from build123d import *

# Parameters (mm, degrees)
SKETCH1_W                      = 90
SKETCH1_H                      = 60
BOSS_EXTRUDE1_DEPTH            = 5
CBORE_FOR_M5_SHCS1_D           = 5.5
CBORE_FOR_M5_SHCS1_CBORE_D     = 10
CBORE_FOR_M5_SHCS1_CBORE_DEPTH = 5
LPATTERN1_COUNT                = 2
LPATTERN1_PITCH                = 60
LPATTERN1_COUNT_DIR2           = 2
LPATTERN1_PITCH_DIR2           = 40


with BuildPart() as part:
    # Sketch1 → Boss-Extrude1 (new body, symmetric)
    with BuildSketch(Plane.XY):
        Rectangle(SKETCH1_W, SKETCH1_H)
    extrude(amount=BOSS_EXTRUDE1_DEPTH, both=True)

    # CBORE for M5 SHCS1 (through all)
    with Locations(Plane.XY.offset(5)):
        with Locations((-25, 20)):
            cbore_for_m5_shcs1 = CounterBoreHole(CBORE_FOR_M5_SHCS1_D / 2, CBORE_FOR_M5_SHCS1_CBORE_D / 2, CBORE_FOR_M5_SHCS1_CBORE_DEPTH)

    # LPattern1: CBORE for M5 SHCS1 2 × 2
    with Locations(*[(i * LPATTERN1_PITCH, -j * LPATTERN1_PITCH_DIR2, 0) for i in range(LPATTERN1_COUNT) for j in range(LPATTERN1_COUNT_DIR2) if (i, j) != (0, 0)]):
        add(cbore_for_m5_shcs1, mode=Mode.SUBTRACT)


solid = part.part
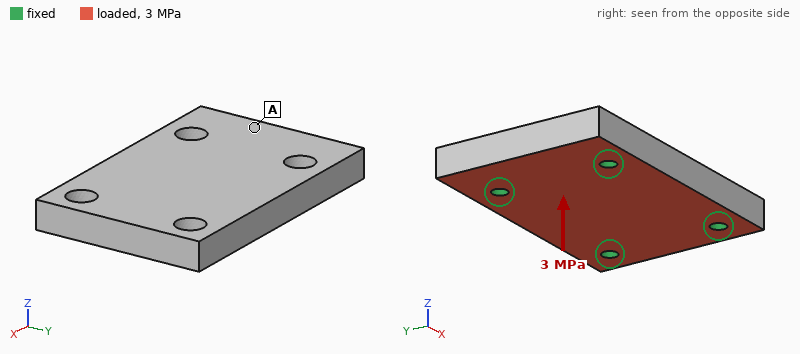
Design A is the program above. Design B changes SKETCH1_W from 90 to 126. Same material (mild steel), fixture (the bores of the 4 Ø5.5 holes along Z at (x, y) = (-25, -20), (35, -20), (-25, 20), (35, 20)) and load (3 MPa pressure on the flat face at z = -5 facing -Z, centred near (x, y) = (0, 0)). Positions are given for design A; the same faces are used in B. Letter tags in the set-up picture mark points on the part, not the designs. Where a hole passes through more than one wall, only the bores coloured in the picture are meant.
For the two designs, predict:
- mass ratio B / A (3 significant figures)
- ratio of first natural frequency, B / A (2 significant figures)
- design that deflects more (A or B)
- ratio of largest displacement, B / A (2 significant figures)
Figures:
1.42
0.46
B
6.1
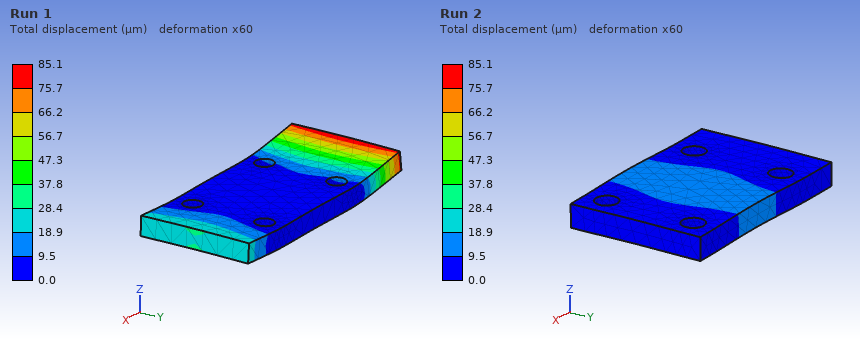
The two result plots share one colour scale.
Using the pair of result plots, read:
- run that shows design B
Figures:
Run 1
